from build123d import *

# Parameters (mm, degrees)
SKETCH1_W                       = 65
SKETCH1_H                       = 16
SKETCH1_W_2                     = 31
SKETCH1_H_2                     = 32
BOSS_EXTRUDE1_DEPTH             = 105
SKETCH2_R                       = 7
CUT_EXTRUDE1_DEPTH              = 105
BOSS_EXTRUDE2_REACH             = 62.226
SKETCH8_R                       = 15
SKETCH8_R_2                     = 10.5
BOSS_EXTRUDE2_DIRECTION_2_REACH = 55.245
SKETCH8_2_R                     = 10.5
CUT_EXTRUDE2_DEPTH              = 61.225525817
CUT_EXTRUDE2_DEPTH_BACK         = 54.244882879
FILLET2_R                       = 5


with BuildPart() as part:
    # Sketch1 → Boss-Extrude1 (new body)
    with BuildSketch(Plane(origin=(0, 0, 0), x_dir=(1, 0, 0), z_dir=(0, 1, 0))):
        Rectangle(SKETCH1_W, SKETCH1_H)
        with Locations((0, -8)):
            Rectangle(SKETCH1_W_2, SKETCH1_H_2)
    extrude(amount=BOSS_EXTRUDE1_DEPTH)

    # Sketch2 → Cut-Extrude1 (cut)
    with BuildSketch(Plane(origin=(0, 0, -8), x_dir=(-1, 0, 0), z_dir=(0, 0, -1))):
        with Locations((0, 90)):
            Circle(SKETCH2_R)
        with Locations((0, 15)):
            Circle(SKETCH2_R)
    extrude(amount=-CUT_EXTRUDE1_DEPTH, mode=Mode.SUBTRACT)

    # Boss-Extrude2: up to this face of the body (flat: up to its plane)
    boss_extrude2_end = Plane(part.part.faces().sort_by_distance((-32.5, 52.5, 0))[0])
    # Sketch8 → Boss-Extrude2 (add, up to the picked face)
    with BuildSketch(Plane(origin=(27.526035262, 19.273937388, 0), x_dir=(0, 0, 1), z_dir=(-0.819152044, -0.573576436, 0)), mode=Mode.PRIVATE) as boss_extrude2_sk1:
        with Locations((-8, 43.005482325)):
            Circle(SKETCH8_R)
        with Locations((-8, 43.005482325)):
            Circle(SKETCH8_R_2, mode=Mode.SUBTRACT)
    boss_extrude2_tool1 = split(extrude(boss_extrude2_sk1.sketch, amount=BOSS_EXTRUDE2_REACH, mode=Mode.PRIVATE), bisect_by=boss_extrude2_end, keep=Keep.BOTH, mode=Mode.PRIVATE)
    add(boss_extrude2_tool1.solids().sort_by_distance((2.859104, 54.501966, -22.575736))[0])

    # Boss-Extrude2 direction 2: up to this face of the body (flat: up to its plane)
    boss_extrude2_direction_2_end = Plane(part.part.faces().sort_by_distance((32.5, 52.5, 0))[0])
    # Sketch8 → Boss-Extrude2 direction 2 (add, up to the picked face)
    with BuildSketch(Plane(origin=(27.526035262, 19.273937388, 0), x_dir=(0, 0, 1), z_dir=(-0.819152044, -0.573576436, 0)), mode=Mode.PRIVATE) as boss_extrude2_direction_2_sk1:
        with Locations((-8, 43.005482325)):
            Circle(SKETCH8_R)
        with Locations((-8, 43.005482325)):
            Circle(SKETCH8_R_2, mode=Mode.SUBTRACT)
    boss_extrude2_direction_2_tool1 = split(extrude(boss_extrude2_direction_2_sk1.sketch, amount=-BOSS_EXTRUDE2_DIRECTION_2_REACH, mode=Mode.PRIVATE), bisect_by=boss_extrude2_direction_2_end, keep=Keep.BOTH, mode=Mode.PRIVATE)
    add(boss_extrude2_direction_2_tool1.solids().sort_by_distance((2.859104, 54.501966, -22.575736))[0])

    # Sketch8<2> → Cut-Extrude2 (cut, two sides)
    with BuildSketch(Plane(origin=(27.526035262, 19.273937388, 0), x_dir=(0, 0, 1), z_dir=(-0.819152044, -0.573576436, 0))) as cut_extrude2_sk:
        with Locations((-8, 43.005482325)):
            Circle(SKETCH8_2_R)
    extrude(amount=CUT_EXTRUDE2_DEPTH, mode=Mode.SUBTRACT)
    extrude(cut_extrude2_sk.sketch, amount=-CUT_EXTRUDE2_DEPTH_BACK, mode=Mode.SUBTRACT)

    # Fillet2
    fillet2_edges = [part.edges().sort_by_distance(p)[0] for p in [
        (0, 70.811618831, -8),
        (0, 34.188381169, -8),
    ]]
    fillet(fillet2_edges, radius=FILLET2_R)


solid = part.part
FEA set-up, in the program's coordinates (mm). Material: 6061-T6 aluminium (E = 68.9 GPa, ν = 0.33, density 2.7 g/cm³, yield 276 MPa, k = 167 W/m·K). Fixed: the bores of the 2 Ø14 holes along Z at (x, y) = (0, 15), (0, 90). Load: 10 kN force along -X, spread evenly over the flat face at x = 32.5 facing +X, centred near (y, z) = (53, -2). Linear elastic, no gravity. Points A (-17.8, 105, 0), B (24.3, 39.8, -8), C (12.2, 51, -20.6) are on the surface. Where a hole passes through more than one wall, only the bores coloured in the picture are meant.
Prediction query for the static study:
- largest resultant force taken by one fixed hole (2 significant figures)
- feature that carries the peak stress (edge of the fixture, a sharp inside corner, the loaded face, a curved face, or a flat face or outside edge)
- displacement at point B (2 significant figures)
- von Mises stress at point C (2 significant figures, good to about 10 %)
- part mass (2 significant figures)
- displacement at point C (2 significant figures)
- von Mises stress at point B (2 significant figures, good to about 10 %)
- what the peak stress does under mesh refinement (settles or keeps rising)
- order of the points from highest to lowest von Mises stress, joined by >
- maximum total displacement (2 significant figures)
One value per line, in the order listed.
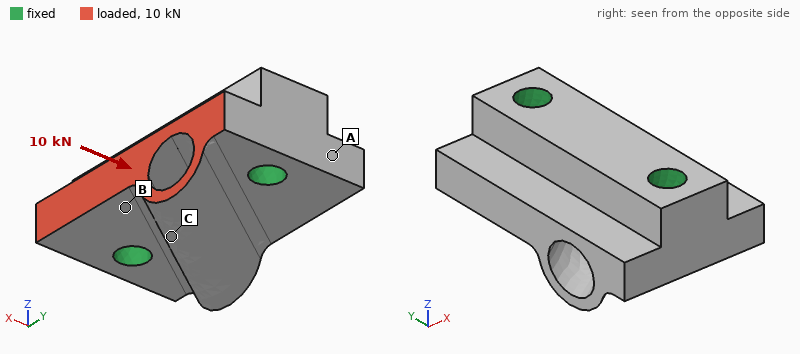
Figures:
5.1 kN
edge of the fixture
6.7 µm
3.7 MPa
410 g
7.2 µm
6.9 MPa
keeps rising
B > C > A
17 µm
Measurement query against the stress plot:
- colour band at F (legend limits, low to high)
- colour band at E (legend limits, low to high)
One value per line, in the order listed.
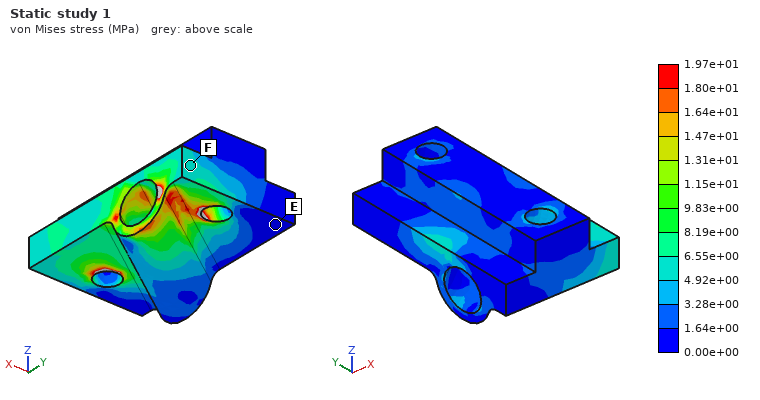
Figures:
4.92e+00 to 6.55e+00 MPa
0.00e+00 to 1.64e+00 MPa
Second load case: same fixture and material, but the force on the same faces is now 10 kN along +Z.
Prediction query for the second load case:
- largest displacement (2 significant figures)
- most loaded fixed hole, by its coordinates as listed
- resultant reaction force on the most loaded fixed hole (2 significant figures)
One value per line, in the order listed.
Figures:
44 µm
(0, 15)
5.4 kN
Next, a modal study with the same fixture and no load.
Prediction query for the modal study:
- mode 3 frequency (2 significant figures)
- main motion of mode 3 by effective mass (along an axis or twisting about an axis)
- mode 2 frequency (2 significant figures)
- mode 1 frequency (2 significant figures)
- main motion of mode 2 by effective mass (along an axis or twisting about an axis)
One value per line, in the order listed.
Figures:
15 kHz
along X
14 kHz
11 kHz
along Z
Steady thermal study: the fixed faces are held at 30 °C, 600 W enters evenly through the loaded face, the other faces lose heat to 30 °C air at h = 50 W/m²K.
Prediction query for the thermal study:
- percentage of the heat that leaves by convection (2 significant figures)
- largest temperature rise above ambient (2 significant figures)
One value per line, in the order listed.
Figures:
4.0 %
82 K
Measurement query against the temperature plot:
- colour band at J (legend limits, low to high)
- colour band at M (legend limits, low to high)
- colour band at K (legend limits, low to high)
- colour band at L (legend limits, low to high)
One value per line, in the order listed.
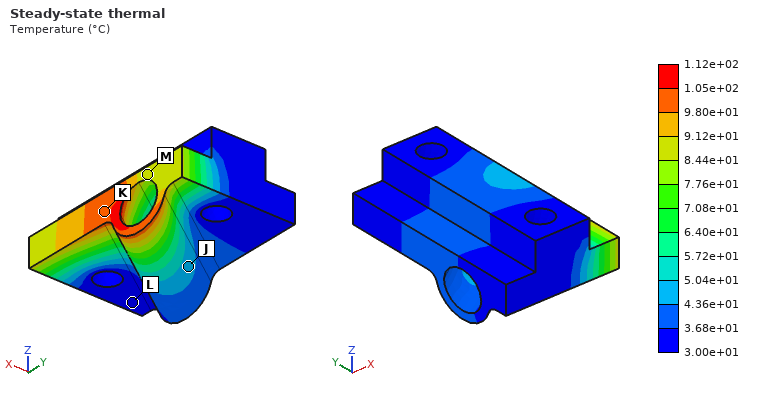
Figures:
4.36e+01 to 5.04e+01 °C
8.44e+01 to 9.12e+01 °C
9.80e+01 to 1.05e+02 °C
3.00e+01 to 3.68e+01 °C
